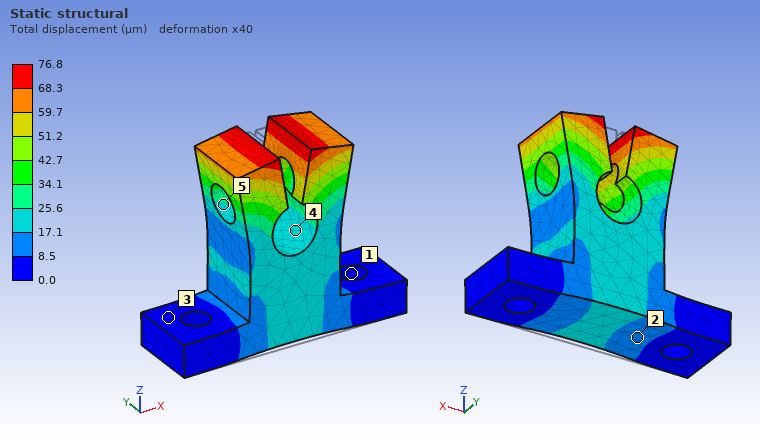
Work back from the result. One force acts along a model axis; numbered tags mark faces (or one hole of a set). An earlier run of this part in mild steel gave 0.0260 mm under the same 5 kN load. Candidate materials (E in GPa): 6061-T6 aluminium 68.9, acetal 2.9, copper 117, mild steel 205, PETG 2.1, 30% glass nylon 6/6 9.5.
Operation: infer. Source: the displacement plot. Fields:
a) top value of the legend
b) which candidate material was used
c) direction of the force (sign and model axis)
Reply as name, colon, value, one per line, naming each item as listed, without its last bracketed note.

top value of the legend: 76.8 µm
which candidate material was used: 6061-T6 aluminium
direction of the force: +Z
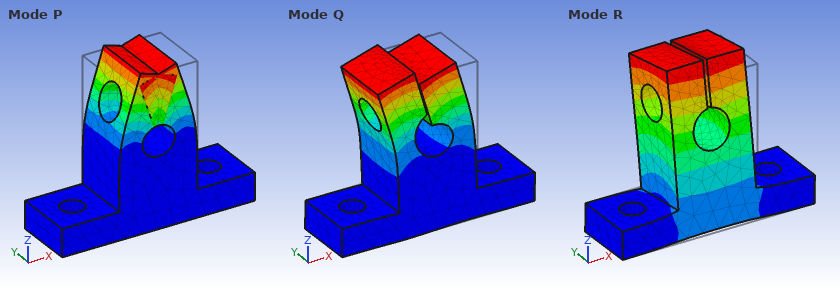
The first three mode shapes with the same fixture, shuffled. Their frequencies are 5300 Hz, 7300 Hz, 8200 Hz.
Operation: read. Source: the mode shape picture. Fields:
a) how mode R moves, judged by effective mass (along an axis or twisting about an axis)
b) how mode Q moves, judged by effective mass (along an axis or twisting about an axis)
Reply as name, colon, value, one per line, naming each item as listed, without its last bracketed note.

how mode R moves, judged by effective mass: along Y
how mode Q moves, judged by effective mass: along X
